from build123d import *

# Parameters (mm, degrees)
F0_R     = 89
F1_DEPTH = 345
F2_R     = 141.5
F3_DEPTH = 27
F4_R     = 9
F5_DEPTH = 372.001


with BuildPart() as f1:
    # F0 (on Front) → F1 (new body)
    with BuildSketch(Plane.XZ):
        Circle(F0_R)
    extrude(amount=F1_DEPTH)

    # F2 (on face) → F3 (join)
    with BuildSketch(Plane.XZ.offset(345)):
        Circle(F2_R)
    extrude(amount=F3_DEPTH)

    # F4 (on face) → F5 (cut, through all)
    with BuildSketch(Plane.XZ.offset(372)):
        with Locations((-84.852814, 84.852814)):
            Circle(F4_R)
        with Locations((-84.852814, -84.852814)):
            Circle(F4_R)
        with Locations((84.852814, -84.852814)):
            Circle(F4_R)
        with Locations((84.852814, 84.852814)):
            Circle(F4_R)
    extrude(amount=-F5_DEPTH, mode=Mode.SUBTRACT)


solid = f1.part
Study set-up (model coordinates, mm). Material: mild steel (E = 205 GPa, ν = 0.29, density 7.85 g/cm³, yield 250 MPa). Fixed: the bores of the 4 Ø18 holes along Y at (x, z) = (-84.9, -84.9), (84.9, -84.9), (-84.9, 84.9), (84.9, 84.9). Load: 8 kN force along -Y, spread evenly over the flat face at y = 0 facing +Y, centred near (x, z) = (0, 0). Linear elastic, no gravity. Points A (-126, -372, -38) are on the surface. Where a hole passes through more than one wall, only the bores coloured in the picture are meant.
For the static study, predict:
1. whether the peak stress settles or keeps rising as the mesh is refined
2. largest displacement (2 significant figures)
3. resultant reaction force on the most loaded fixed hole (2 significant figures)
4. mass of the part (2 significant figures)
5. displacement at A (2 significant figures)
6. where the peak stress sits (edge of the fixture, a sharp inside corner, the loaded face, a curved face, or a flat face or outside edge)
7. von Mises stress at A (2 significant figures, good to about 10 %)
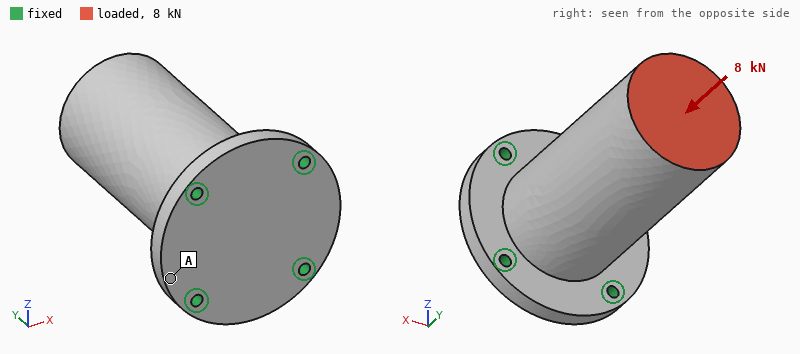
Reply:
keeps rising
1.7 µm
2.1 kN
81 kg
0.62 µm
edge of the fixture
0.76 MPa
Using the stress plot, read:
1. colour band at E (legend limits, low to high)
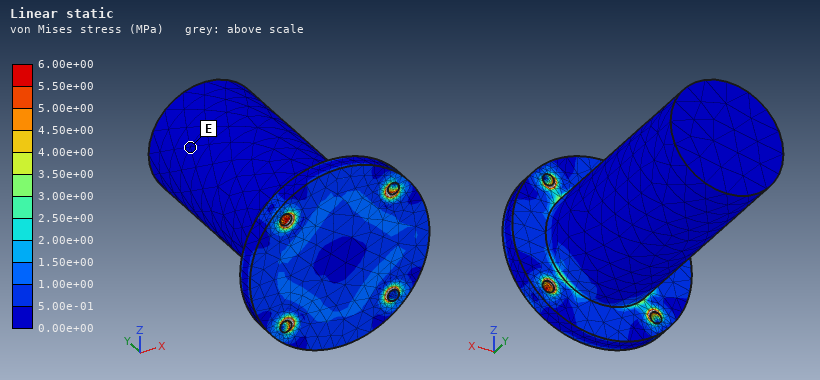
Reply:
0.00e+00 to 5.00e-01 MPa
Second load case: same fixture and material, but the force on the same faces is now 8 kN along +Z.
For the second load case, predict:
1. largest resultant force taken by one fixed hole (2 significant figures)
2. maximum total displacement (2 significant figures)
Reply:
9.4 kN
40 µm
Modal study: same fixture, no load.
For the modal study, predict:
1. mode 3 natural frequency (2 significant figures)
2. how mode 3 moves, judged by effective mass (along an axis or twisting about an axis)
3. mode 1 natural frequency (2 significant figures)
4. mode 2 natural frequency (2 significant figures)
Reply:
1400 Hz
along Y
490 Hz
490 Hz
